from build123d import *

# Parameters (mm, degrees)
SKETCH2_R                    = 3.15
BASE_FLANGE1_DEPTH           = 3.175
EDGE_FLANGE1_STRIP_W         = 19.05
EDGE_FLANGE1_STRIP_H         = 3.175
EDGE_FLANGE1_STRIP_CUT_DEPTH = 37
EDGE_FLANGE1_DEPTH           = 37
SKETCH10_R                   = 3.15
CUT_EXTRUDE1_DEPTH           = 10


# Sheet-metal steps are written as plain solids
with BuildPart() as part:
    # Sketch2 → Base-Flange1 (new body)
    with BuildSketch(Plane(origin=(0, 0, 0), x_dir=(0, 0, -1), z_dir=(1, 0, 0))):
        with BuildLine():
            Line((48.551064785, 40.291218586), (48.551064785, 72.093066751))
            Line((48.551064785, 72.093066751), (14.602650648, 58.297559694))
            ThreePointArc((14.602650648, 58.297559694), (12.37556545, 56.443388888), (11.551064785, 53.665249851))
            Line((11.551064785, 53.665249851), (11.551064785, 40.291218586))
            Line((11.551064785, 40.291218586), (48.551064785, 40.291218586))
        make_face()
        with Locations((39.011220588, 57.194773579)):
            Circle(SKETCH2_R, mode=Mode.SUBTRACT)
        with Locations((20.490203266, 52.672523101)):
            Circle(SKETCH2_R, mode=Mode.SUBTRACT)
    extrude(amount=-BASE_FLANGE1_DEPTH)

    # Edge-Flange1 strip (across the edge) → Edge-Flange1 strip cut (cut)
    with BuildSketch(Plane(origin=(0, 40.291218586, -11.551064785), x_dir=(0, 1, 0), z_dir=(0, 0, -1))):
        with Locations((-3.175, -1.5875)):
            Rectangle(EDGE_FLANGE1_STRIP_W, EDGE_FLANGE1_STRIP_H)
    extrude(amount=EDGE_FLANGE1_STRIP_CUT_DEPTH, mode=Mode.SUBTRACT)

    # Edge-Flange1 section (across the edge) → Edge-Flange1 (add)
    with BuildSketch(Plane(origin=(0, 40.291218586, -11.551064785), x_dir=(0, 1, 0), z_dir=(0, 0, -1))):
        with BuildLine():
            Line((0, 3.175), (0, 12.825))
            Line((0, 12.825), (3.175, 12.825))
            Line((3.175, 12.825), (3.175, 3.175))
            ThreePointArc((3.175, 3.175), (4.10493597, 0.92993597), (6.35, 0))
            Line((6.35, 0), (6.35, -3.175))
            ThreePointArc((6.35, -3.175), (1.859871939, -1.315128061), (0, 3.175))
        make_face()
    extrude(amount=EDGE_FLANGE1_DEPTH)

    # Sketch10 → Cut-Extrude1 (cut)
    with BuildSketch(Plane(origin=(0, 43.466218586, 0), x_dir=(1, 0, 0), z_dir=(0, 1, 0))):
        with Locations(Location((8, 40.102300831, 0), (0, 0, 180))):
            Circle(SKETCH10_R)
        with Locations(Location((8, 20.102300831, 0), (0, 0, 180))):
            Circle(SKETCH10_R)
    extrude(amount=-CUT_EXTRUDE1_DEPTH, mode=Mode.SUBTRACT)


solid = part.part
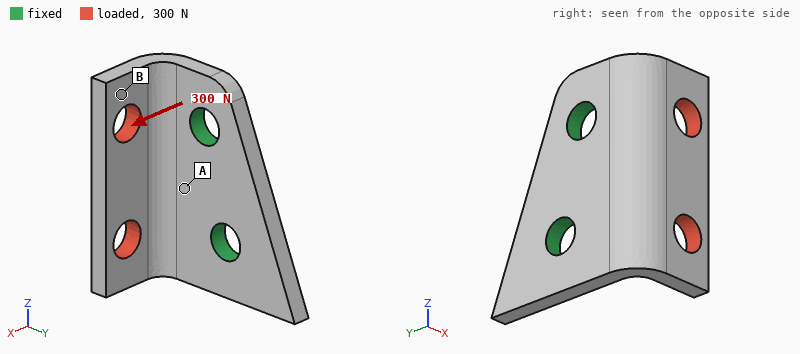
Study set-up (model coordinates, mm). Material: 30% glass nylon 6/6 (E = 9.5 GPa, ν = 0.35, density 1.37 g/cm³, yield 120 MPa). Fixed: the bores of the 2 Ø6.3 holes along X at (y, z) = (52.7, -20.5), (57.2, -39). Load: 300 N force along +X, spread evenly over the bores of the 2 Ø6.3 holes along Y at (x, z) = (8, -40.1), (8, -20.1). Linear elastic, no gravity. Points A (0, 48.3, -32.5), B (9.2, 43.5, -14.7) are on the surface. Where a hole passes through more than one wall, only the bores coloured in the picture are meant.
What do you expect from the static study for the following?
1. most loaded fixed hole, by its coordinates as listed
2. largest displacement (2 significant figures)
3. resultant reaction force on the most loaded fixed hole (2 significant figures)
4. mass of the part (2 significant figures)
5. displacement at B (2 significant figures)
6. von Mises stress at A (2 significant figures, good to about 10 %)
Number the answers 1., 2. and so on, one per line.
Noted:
1. (52.7, -20.5)
2. 0.41 mm
3. 190 N
4. 5.1 g
5. 0.18 mm
6. 23 MPa
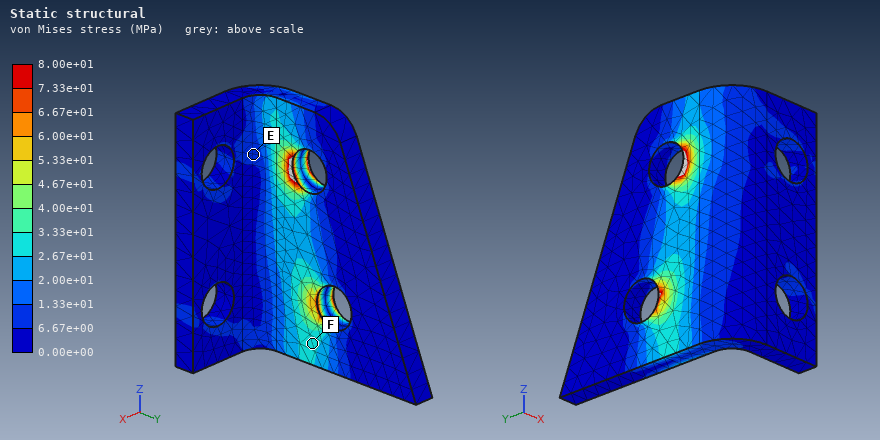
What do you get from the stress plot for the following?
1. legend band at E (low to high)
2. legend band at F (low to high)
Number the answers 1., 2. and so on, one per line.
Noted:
1. 6.67e+00 to 1.33e+01 MPa
2. 2.67e+01 to 3.33e+01 MPa
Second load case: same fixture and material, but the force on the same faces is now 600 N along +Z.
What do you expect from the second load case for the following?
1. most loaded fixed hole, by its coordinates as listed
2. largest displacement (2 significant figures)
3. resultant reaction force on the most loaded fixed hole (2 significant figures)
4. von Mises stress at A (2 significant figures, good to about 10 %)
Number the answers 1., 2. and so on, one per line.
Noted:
1. (52.7, -20.5)
2. 0.52 mm
3. 540 N
4. 35 MPa
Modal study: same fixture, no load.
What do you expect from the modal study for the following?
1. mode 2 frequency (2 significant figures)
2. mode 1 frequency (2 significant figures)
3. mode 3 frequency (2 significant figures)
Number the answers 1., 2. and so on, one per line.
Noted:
1. 4700 Hz
2. 3100 Hz
3. 7800 Hz
